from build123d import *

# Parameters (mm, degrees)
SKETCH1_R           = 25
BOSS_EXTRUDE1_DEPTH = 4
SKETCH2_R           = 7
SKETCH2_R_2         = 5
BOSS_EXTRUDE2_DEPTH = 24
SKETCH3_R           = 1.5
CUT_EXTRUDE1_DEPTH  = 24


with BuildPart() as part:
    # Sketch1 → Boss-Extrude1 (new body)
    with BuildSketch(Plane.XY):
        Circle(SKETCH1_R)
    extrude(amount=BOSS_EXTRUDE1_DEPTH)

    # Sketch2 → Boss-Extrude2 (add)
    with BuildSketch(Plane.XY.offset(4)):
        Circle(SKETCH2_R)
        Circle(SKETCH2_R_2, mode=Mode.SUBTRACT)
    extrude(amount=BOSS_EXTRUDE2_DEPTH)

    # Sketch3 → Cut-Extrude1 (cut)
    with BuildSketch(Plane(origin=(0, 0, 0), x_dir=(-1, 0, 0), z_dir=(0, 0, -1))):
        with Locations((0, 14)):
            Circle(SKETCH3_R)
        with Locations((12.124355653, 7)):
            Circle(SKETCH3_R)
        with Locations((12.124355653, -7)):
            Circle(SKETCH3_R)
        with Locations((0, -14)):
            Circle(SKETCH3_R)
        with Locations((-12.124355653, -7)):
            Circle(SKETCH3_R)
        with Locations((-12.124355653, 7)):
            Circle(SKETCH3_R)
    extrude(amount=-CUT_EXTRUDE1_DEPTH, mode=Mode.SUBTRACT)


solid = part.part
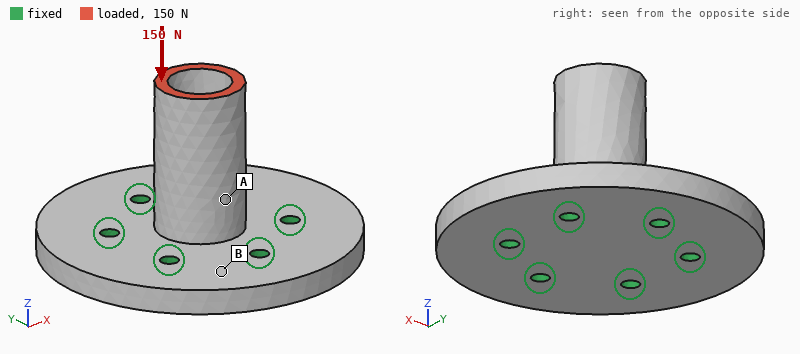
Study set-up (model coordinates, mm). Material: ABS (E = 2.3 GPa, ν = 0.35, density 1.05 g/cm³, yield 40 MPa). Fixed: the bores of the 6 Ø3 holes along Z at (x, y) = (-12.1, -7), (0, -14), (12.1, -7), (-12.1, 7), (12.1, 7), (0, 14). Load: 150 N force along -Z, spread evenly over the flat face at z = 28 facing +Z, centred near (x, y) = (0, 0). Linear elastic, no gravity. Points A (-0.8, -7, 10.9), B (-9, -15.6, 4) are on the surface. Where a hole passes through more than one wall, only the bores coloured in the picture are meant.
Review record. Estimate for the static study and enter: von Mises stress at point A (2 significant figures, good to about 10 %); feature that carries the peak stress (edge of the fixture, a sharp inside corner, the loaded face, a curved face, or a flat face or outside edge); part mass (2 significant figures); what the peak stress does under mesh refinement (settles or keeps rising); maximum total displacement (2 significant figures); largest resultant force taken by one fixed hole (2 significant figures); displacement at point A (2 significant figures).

1.7 MPa
edge of the fixture
10.0 g
keeps rising
38 µm
26 N
23 µm
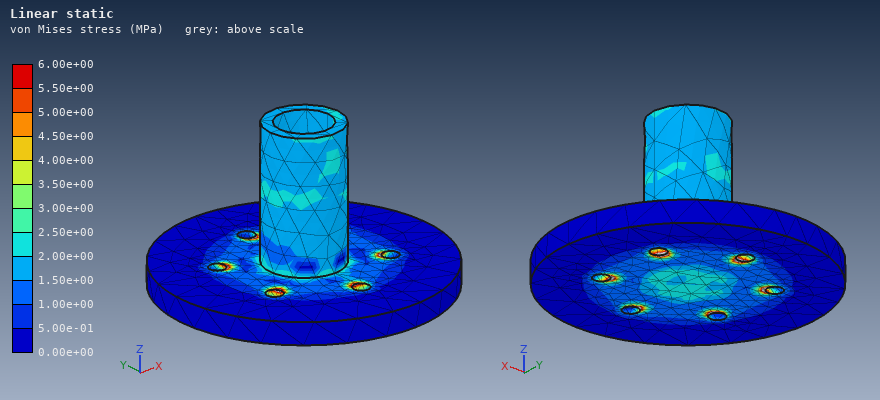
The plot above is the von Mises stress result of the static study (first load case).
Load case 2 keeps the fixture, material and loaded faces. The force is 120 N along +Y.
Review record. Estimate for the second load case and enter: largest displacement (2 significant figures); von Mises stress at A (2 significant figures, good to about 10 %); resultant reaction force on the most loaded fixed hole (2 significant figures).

0.45 mm
9.6 MPa
97 N
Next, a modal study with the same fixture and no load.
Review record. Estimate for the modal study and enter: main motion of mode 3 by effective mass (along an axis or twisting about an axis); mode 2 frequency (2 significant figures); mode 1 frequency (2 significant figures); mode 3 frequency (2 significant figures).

along Z
3400 Hz
3400 Hz
6300 Hz
